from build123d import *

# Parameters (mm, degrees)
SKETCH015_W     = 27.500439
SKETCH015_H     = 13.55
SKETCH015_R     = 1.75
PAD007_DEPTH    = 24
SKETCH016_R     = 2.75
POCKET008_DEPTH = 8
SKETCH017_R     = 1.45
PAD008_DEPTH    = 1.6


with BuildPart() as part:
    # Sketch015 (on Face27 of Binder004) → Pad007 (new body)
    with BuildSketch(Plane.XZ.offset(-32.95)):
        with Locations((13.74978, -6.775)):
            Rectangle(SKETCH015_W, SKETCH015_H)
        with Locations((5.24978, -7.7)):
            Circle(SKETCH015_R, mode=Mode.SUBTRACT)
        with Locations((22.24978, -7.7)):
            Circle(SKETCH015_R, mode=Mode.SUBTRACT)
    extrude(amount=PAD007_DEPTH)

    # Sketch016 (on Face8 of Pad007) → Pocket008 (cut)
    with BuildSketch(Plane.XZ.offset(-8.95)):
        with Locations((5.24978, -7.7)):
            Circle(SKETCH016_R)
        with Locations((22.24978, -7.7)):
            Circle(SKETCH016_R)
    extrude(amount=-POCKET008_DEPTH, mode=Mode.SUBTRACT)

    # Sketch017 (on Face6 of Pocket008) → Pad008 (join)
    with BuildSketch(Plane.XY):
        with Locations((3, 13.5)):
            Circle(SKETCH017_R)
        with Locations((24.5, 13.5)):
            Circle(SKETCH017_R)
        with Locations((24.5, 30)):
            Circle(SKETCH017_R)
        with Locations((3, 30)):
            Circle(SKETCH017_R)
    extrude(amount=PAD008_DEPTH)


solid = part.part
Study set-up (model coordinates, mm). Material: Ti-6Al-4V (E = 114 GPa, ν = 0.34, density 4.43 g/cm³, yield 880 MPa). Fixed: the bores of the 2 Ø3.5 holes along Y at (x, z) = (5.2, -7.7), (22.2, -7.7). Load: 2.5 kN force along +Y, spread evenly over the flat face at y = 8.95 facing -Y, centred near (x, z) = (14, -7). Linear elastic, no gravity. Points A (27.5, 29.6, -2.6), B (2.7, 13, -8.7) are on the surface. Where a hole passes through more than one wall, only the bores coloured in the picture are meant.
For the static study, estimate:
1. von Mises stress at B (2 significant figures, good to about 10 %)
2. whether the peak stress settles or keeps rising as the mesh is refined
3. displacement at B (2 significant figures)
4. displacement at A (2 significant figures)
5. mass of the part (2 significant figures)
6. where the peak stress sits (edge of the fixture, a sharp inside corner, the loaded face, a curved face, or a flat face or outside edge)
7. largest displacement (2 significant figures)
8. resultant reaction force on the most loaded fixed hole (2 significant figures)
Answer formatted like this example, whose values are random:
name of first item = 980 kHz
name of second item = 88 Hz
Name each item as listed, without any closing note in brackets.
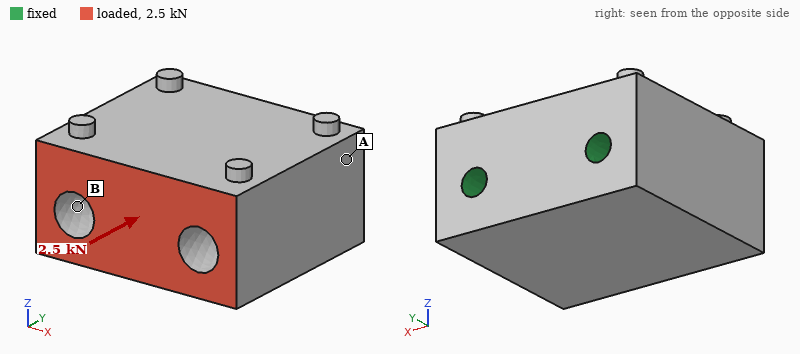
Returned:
von Mises stress at B = 9.7 MPa
whether the peak stress settles or keeps rising as the mesh is refined = keeps rising
displacement at B = 0.81 µm
displacement at A = 0.30 µm
mass of the part = 37 g
where the peak stress sits = edge of the fixture
largest displacement = 1.4 µm
resultant reaction force on the most loaded fixed hole = 1.3 kN
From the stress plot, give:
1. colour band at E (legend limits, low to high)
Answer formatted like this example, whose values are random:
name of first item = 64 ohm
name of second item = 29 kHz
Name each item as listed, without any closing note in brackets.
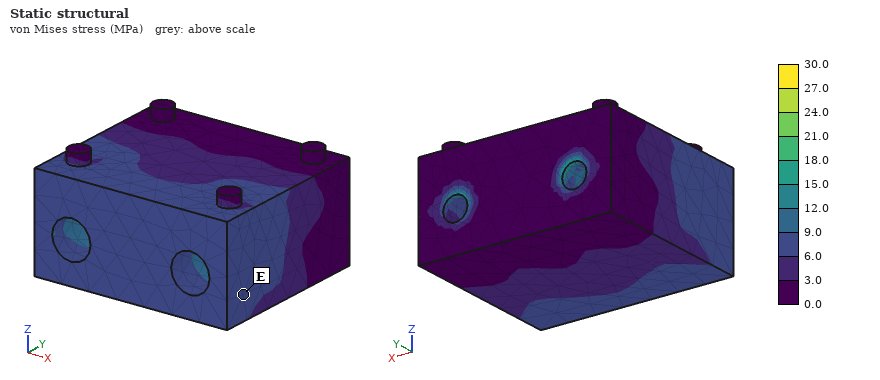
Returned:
colour band at E = 6.0 to 9.0 MPa
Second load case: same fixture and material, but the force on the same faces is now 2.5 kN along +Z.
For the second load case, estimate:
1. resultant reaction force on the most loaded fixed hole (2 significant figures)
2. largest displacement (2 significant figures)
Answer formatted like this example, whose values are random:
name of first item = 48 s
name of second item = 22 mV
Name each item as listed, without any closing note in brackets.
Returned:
resultant reaction force on the most loaded fixed hole = 1.3 kN
largest displacement = 9.7 µm
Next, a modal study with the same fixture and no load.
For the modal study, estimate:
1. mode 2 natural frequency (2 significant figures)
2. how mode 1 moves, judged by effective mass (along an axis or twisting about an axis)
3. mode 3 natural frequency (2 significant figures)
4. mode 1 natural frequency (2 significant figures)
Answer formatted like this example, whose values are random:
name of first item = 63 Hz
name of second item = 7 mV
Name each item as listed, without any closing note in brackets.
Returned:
mode 2 natural frequency = 49 kHz
how mode 1 moves, judged by effective mass = along Z
mode 3 natural frequency = 49 kHz
mode 1 natural frequency = 34 kHz
